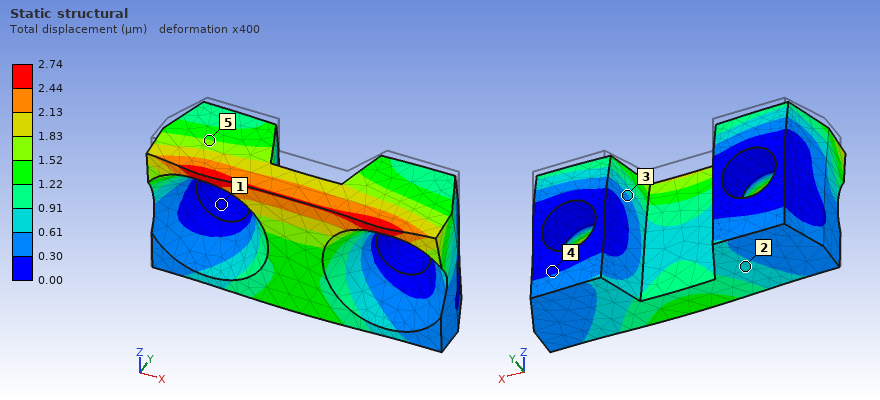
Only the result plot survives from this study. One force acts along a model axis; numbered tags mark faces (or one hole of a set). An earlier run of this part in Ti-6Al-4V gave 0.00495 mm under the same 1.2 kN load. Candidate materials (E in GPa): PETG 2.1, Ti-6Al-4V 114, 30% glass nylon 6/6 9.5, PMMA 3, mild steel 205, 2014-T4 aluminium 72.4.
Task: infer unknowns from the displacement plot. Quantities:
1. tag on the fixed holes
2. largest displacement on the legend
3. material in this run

1
2.74 µm
mild steel
